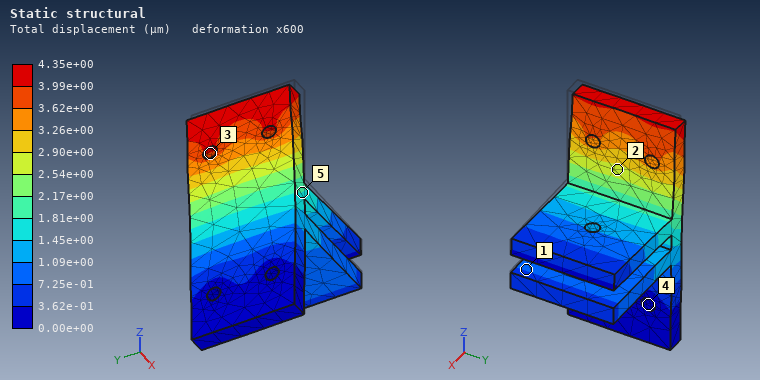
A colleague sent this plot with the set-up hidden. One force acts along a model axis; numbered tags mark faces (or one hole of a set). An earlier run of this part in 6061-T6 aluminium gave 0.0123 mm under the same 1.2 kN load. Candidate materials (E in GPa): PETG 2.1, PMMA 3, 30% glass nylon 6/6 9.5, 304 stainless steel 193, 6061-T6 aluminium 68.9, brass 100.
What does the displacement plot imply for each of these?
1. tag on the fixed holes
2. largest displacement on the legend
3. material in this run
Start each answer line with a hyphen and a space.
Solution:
- 4
- 4.35e+00 µm
- 304 stainless steel
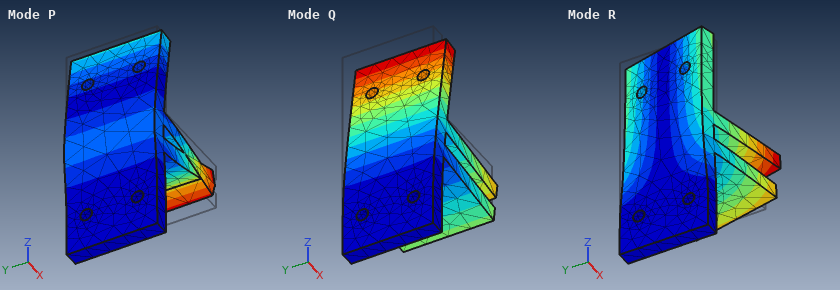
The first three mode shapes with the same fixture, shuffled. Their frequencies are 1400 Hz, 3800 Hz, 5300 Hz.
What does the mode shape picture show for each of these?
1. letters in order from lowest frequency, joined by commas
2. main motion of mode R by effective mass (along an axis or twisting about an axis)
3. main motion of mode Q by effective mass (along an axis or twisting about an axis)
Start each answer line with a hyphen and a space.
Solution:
- Q, R, P
- along Y
- along X
